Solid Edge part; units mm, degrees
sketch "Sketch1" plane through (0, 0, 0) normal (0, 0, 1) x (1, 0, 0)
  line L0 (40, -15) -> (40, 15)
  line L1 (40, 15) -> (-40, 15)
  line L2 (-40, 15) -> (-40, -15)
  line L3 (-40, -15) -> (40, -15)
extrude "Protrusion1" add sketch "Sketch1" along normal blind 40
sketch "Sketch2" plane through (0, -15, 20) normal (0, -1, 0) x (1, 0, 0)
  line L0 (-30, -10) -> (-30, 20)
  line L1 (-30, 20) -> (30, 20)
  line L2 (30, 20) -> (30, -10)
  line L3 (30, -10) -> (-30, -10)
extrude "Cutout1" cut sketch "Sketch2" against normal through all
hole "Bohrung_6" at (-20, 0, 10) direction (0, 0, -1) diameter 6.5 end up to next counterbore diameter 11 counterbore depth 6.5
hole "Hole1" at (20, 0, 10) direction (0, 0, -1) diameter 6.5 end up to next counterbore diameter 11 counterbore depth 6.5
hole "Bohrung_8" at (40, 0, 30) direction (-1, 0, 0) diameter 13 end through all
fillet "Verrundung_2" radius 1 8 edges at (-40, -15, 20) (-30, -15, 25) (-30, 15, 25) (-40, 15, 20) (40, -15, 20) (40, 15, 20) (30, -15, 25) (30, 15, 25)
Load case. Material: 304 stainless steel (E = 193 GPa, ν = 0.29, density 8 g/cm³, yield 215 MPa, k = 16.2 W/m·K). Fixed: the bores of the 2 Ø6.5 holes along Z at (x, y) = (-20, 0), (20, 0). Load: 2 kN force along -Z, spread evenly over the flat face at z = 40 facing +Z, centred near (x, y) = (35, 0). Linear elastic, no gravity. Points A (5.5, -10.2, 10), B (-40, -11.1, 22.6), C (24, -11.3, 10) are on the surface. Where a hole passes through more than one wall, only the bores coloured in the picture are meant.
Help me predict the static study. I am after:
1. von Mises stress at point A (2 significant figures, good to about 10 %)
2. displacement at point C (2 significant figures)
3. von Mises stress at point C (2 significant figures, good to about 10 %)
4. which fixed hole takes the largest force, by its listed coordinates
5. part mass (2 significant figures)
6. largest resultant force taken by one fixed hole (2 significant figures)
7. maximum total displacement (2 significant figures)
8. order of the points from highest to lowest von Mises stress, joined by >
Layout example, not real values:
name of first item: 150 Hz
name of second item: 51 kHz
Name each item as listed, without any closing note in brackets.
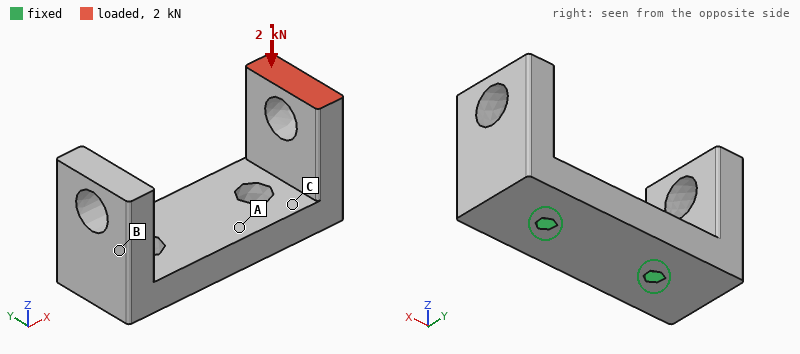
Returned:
von Mises stress at point A: 22 MPa
displacement at point C: 6.5 µm
von Mises stress at point C: 48 MPa
which fixed hole takes the largest force, by its listed coordinates: (20, 0)
part mass: 300 g
largest resultant force taken by one fixed hole: 2.8 kN
maximum total displacement: 43 µm
order of the points from highest to lowest von Mises stress, joined by >: C > A > B
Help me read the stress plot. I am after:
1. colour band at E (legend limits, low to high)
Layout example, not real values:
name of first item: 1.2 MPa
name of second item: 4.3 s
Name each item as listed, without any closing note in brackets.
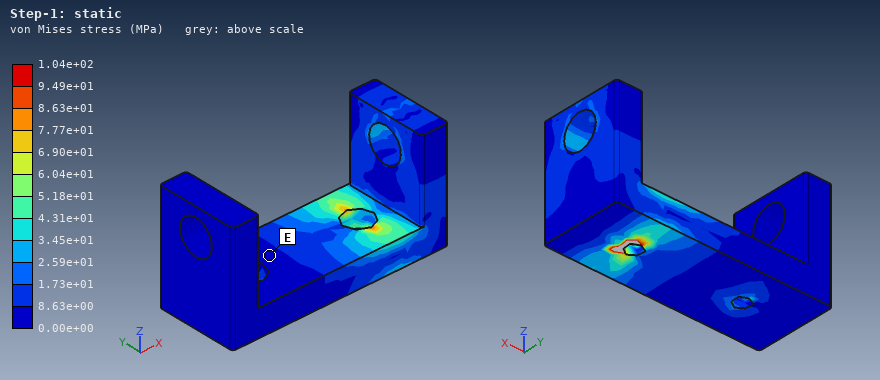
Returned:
colour band at E: 0.00e+00 to 8.63e+00 MPa
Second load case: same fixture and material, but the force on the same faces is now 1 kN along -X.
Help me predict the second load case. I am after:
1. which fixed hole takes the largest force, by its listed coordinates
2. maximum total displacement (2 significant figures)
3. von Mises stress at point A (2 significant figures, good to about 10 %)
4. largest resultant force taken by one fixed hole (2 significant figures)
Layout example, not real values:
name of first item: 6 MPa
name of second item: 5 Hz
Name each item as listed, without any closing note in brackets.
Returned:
which fixed hole takes the largest force, by its listed coordinates: (-20, 0)
maximum total displacement: 99 µm
von Mises stress at point A: 30 MPa
largest resultant force taken by one fixed hole: 2.1 kN
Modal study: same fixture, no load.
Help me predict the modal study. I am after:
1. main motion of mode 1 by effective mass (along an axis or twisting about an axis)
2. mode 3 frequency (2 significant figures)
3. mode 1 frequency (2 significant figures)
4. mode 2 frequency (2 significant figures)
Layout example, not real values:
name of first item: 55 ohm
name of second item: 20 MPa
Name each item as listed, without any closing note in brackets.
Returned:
main motion of mode 1 by effective mass: along Y
mode 3 frequency: 3300 Hz
mode 1 frequency: 2700 Hz
mode 2 frequency: 3300 Hz
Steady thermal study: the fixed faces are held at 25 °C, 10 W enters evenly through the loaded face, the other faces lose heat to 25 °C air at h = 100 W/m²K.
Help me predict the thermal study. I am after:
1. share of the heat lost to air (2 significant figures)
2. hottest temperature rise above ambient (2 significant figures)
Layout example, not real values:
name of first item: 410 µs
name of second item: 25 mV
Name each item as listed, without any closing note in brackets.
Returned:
share of the heat lost to air: 85 %
hottest temperature rise above ambient: 62 K
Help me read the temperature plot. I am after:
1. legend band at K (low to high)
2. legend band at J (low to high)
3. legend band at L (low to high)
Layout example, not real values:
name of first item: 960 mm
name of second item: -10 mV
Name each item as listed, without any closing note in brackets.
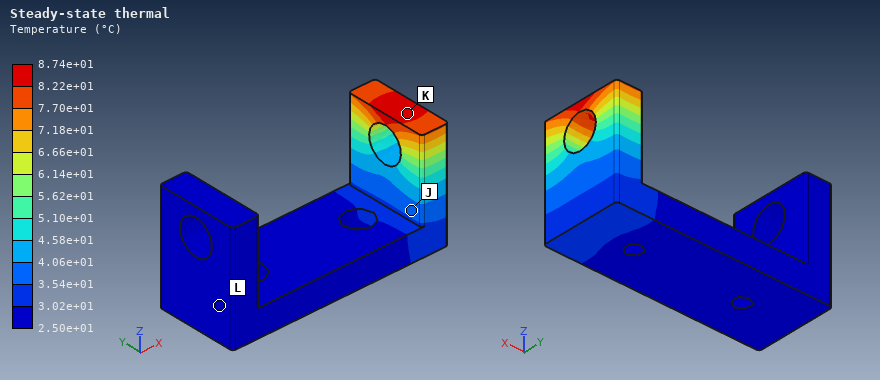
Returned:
legend band at K: 8.22e+01 to 8.74e+01 °C
legend band at J: 3.54e+01 to 4.06e+01 °C
legend band at L: 2.50e+01 to 3.02e+01 °C
